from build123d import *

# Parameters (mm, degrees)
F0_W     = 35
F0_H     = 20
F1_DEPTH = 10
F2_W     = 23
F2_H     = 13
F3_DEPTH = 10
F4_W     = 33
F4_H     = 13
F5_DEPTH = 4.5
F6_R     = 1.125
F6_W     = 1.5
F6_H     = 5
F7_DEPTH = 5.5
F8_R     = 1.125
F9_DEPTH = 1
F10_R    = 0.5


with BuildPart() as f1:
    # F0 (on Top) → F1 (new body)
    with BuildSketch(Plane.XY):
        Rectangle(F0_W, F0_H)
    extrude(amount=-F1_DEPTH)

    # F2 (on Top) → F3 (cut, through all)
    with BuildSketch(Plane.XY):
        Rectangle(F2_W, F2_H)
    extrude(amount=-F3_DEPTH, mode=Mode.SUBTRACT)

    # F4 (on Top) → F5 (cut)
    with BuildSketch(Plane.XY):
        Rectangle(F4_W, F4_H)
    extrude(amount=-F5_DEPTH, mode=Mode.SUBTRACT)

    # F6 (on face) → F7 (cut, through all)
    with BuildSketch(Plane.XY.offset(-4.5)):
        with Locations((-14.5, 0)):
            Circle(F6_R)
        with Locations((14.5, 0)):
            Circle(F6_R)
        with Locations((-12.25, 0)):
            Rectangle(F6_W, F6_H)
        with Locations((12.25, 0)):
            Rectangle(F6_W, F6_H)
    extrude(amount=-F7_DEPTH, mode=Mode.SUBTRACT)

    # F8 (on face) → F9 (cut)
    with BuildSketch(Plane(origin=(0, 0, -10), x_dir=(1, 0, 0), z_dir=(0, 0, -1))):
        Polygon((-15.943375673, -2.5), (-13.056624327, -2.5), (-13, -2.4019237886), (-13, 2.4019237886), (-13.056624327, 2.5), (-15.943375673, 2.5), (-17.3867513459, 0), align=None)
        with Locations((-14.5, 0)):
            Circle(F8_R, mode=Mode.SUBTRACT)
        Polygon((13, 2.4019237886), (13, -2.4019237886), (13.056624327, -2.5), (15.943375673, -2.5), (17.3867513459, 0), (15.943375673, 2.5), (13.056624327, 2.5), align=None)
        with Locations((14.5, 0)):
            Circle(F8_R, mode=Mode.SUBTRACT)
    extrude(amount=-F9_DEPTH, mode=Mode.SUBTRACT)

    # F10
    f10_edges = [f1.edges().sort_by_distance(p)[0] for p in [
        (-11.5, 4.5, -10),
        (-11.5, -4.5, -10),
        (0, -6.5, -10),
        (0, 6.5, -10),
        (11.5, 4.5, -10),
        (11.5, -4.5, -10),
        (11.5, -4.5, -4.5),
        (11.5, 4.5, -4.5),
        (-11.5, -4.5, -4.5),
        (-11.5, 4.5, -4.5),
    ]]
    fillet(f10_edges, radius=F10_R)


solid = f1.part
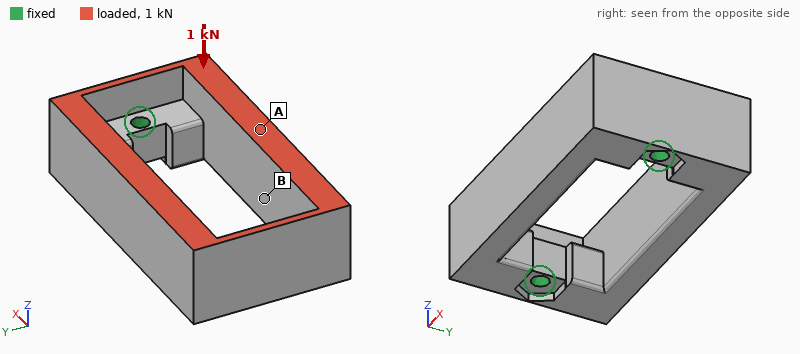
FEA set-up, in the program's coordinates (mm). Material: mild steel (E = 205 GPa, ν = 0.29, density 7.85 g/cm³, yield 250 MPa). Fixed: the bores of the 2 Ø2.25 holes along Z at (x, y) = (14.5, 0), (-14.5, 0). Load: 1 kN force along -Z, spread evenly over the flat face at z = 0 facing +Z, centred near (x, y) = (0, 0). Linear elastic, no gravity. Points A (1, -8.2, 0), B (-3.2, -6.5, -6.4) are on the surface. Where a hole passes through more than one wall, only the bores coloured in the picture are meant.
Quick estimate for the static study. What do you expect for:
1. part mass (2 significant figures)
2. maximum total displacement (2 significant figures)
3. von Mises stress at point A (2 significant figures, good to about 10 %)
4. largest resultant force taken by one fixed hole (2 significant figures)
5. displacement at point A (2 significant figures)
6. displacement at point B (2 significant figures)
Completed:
26 g
6.4 µm
19 MPa
500 N
5.8 µm
4.2 µm
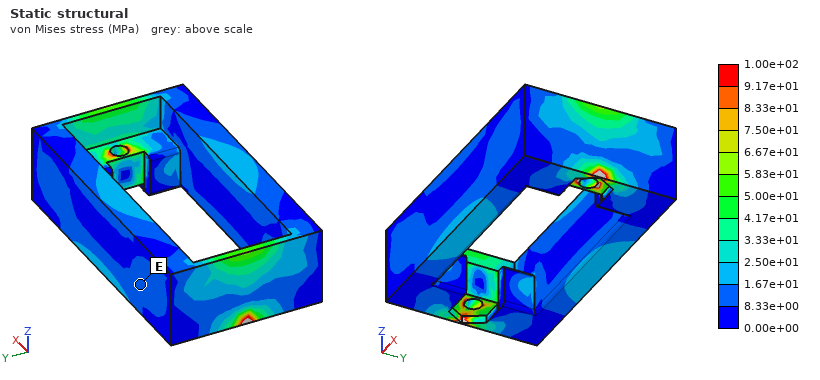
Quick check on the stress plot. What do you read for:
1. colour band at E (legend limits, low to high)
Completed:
8.33e+00 to 1.67e+01 MPa
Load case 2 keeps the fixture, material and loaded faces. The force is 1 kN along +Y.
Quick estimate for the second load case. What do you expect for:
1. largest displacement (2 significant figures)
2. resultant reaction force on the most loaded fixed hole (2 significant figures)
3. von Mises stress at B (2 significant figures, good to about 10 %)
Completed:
18 µm
500 N
21 MPa
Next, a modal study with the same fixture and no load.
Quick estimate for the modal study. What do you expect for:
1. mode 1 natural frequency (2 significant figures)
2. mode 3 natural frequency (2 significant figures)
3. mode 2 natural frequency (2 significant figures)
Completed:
12 kHz
16 kHz
15 kHz
